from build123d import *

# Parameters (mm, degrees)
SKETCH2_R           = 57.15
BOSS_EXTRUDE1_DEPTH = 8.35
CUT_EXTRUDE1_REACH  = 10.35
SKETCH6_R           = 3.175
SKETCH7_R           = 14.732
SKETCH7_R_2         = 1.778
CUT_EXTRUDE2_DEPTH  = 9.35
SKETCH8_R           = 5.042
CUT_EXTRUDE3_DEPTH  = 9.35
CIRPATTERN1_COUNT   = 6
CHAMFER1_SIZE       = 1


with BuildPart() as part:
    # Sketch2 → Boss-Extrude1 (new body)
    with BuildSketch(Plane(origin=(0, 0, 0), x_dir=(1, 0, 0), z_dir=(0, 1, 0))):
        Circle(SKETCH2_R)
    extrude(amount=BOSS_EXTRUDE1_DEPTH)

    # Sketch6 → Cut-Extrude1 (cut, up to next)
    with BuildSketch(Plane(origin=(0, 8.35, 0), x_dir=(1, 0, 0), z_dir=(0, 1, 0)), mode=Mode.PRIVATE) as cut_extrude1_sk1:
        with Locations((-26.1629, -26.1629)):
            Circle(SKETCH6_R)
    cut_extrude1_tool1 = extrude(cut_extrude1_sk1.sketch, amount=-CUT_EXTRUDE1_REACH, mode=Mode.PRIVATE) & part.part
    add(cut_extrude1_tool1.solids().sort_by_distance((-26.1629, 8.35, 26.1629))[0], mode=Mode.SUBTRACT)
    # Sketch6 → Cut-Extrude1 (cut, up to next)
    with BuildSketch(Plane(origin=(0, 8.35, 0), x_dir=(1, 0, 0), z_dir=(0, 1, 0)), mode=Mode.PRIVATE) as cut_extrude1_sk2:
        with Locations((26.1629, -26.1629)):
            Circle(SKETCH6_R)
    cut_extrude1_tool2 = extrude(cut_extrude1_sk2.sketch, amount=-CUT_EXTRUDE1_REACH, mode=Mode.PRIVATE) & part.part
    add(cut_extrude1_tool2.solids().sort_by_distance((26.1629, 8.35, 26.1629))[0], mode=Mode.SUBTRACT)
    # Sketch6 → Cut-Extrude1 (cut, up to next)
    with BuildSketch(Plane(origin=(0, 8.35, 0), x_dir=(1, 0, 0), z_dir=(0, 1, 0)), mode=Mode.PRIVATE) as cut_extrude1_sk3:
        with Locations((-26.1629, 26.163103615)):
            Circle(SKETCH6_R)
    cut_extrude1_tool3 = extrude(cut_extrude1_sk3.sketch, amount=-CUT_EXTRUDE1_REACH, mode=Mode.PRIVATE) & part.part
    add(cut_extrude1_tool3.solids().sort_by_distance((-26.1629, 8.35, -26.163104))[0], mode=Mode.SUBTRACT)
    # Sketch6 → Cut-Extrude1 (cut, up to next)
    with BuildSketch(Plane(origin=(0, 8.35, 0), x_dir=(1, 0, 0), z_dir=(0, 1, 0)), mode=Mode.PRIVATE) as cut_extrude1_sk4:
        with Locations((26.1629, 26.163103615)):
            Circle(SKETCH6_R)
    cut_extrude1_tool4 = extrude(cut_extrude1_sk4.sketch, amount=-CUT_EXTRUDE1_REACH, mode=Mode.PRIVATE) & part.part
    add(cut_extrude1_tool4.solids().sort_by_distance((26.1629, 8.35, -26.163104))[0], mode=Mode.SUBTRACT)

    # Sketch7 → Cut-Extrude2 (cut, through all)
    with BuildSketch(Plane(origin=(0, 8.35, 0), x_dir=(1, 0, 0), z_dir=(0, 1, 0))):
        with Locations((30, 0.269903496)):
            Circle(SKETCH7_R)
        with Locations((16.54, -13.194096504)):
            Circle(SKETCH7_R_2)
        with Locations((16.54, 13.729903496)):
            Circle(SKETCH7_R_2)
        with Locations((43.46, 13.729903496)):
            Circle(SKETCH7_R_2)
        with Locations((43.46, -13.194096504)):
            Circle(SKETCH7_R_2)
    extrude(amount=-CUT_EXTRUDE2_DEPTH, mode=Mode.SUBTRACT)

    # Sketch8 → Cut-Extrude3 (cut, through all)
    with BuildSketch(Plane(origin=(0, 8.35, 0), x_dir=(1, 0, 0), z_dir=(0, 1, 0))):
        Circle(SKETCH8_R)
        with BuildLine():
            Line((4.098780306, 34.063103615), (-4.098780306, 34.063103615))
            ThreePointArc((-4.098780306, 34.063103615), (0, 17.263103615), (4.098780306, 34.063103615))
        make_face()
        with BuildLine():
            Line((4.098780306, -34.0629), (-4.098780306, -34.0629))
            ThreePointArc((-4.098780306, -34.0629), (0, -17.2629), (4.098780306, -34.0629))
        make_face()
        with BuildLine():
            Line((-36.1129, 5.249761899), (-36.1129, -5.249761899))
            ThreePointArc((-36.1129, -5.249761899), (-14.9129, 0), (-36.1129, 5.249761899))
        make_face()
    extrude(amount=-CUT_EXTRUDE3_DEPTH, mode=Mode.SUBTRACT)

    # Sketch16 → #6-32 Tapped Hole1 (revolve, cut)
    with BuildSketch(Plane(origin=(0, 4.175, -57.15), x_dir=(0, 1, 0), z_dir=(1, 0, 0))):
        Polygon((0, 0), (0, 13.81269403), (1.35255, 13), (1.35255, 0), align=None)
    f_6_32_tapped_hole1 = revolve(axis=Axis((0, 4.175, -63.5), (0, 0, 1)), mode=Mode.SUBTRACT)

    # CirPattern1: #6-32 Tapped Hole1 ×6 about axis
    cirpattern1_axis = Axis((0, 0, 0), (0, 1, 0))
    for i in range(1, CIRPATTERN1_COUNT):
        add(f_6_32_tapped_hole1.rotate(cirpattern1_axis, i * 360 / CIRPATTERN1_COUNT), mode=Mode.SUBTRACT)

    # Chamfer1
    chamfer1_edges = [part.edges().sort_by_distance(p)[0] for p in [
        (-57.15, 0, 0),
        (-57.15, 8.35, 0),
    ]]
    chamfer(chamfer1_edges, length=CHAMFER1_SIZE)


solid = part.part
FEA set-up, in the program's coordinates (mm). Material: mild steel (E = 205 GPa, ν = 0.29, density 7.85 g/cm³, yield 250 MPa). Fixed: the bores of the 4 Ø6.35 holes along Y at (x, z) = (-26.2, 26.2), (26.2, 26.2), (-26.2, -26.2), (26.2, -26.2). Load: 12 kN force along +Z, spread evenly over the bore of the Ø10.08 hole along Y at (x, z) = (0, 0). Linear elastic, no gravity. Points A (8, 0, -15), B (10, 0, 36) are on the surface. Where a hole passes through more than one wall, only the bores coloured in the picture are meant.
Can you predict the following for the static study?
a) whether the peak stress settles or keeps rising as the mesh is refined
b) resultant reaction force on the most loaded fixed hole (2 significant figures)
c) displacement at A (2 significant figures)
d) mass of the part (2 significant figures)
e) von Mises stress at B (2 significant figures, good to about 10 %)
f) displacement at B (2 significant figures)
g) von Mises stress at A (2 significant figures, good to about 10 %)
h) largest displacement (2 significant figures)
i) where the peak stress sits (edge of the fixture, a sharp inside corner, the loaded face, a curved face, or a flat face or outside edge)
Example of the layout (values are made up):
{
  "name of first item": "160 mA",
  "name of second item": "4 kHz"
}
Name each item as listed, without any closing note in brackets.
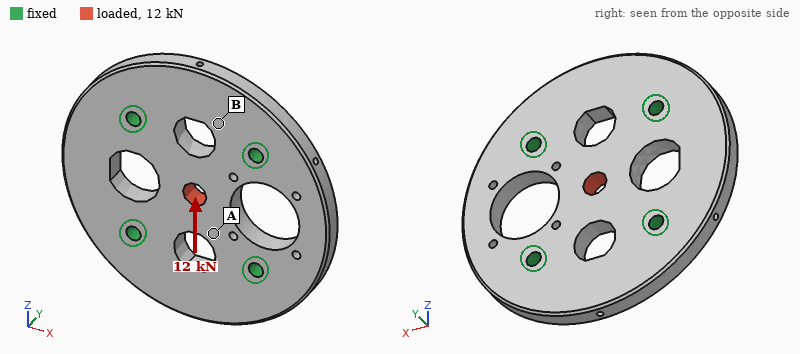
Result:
{
  "whether the peak stress settles or keeps rising as the mesh is refined": "keeps rising",
  "resultant reaction force on the most loaded fixed hole": "3.4 kN",
  "displacement at A": "3.6 µm",
  "mass of the part": "550 g",
  "von Mises stress at B": "9.0 MPa",
  "displacement at B": "1.4 µm",
  "von Mises stress at A": "29 MPa",
  "largest displacement": "6.0 µm",
  "where the peak stress sits": "a sharp inside corner"
}
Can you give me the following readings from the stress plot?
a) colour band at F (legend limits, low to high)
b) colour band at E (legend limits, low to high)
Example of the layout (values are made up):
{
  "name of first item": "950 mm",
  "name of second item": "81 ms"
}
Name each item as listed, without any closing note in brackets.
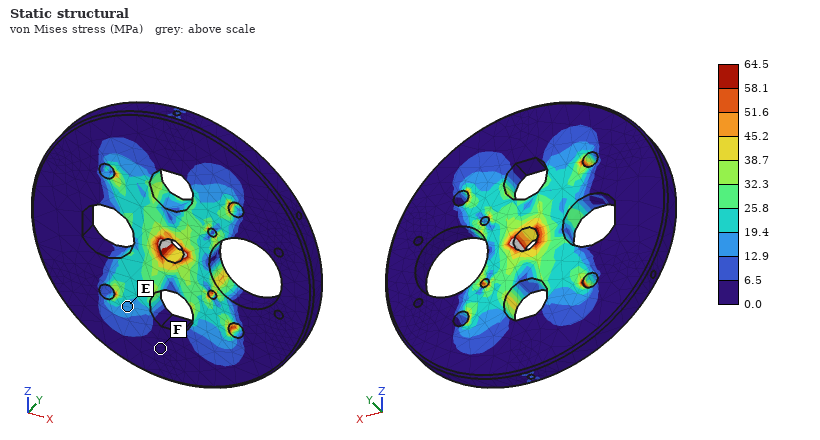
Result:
{
  "colour band at F": "0.0 to 6.5 MPa",
  "colour band at E": "12.9 to 19.4 MPa"
}
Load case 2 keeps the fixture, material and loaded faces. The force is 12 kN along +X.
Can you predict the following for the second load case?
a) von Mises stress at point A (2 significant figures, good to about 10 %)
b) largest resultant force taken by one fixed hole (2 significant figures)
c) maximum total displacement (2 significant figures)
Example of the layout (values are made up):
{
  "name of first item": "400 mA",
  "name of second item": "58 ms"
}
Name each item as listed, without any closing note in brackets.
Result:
{
  "von Mises stress at point A": "23 MPa",
  "largest resultant force taken by one fixed hole": "3.7 kN",
  "maximum total displacement": "7.0 µm"
}
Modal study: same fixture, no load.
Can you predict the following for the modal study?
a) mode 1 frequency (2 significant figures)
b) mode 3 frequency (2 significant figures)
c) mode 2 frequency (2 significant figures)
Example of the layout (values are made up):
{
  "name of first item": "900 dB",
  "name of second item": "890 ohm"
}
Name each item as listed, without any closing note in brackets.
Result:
{
  "mode 1 frequency": "6200 Hz",
  "mode 3 frequency": "7000 Hz",
  "mode 2 frequency": "6700 Hz"
}
